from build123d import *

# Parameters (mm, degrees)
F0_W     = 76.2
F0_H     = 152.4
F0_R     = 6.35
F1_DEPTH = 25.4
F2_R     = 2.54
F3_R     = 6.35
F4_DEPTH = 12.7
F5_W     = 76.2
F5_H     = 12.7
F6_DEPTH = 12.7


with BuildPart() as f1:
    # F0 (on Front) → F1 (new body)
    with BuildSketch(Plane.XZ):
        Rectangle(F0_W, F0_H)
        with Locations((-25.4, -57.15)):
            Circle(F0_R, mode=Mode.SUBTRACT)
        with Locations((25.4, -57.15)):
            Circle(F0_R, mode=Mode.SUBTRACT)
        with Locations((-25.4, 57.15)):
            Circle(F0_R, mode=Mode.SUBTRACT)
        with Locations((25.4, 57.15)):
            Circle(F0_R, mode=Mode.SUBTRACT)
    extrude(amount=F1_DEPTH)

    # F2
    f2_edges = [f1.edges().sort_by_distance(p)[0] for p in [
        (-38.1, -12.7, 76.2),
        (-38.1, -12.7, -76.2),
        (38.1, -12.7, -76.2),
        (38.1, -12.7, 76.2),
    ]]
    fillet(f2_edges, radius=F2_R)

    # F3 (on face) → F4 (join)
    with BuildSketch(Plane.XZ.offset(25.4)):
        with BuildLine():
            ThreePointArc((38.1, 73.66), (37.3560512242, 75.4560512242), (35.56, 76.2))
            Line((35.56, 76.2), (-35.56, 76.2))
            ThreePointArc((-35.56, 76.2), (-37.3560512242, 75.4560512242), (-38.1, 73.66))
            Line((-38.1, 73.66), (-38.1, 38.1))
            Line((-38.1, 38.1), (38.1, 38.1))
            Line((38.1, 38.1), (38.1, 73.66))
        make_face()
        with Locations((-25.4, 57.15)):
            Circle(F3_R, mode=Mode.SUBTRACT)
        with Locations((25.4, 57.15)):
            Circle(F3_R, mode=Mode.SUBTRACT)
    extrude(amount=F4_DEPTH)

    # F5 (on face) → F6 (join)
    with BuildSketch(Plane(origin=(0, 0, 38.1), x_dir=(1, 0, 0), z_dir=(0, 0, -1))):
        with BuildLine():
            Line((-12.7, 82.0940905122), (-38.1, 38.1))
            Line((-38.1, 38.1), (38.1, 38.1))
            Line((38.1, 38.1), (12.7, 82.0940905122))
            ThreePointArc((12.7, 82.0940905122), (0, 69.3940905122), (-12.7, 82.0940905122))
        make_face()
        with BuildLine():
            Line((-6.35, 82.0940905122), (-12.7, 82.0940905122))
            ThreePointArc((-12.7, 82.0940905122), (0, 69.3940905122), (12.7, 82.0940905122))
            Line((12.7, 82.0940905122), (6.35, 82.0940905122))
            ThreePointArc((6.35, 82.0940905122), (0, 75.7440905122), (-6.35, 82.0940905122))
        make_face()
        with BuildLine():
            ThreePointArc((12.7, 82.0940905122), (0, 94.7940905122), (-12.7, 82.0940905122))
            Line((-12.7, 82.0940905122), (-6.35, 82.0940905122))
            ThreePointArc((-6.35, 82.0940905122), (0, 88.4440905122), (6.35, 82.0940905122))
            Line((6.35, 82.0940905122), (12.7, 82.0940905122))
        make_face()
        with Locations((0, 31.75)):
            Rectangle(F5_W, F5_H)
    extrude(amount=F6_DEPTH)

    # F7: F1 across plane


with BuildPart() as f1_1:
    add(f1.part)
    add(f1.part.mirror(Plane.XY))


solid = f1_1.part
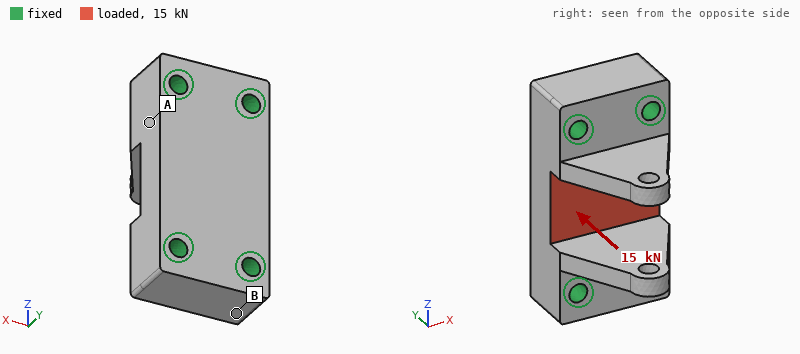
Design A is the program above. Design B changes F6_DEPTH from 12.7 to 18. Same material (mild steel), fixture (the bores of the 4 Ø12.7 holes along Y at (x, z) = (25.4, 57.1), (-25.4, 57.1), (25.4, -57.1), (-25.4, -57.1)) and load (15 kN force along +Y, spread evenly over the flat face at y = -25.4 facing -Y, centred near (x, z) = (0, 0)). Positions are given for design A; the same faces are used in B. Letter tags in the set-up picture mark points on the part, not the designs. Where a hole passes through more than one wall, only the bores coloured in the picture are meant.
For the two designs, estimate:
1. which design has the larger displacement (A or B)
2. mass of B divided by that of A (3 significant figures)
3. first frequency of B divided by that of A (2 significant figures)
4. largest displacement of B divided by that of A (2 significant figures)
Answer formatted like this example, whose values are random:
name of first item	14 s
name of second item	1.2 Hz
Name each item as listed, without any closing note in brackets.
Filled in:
which design has the larger displacement	B
mass of B divided by that of A	1.08
first frequency of B divided by that of A	1.2
largest displacement of B divided by that of A	1.2
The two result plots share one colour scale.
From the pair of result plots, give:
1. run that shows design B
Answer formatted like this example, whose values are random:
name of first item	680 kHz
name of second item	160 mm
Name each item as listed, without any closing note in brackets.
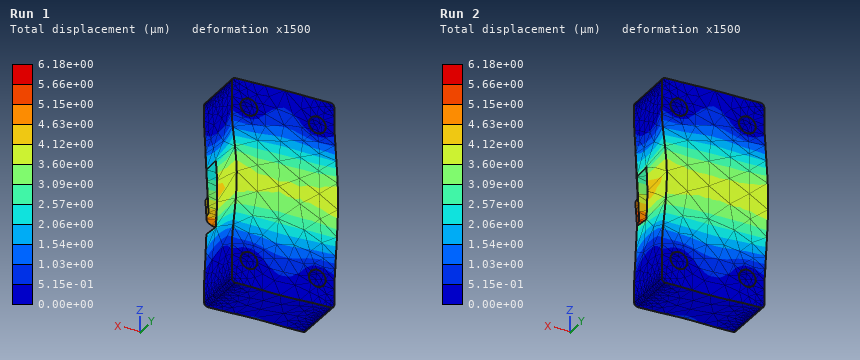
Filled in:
run that shows design B	Run 2
